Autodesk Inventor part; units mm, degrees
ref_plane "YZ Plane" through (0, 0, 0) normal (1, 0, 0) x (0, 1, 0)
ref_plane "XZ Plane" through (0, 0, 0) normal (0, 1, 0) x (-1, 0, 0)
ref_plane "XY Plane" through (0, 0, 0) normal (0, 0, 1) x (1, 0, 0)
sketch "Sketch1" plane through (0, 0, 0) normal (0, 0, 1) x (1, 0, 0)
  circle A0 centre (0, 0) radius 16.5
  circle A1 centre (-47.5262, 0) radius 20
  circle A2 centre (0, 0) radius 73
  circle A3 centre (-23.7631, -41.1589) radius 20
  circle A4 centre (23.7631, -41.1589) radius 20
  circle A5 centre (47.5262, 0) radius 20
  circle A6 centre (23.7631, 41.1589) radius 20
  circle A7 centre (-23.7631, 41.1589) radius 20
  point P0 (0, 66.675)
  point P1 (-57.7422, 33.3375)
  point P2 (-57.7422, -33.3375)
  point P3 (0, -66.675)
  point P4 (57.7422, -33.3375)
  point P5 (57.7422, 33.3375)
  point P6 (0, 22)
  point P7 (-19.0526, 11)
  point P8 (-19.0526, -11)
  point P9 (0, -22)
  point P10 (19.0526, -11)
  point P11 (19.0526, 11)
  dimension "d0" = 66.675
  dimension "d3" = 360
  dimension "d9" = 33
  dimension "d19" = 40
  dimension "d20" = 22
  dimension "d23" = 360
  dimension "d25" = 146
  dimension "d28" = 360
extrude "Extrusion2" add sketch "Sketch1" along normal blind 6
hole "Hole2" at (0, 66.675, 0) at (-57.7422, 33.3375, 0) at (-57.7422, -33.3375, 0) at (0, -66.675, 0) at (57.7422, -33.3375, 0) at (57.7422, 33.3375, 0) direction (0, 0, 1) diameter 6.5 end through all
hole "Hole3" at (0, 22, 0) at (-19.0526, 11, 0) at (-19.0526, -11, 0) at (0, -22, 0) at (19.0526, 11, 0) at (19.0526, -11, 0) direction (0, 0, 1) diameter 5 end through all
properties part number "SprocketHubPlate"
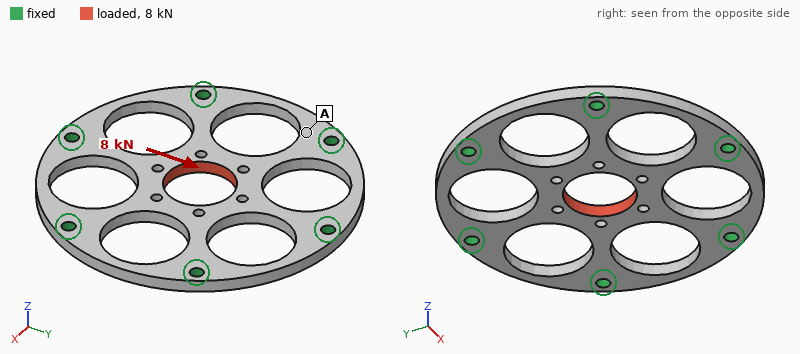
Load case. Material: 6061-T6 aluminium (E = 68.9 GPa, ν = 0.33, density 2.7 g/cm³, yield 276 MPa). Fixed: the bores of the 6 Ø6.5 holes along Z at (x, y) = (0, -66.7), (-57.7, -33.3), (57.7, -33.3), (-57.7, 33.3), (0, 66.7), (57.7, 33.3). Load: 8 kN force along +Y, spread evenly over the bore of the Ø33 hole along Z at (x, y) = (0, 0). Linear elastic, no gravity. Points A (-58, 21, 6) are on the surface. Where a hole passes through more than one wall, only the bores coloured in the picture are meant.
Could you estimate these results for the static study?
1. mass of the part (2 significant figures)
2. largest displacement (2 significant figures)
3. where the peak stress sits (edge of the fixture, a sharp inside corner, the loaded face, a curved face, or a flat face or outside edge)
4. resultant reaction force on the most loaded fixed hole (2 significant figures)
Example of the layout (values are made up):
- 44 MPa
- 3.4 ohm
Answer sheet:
- 130 g
- 26 µm
- a curved face
- 2.3 kN
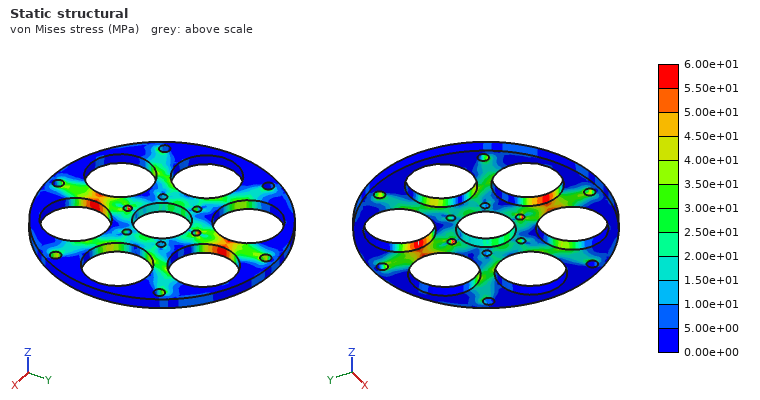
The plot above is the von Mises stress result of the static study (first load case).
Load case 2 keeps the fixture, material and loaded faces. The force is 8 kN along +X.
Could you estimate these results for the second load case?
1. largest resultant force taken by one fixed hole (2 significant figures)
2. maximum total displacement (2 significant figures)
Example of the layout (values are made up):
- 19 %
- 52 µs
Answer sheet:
- 2.0 kN
- 26 µm
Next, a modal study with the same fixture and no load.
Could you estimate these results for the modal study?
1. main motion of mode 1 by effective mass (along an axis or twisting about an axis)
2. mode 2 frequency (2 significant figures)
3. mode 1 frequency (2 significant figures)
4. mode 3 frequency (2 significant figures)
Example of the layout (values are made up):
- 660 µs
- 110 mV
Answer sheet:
- along Z
- 5100 Hz
- 2600 Hz
- 5100 Hz
